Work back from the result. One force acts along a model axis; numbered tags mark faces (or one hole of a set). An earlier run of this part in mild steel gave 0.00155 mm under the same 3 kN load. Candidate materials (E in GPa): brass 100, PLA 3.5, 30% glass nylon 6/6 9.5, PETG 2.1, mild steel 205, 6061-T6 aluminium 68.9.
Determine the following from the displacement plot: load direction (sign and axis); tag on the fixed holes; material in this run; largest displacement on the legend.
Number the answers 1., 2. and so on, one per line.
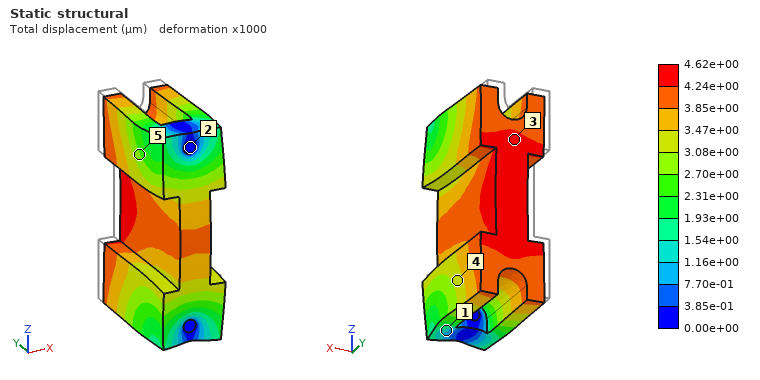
1. -Y
2. 2
3. 6061-T6 aluminium
4. 4.62e+00 µm
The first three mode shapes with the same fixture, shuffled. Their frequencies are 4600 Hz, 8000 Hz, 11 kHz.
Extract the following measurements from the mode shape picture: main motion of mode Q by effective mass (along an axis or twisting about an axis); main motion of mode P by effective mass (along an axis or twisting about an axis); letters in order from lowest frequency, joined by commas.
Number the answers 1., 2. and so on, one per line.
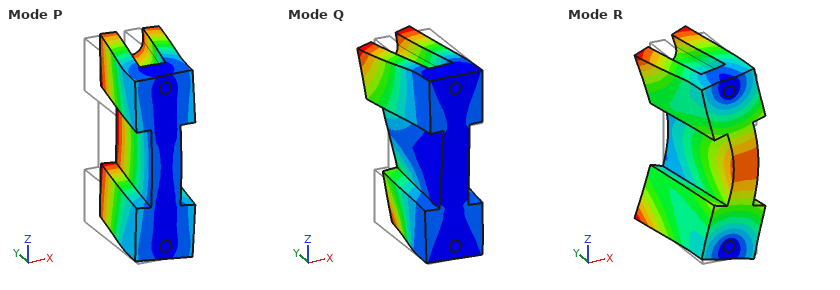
1. twisting about Y
2. along X
3. P, Q, R
